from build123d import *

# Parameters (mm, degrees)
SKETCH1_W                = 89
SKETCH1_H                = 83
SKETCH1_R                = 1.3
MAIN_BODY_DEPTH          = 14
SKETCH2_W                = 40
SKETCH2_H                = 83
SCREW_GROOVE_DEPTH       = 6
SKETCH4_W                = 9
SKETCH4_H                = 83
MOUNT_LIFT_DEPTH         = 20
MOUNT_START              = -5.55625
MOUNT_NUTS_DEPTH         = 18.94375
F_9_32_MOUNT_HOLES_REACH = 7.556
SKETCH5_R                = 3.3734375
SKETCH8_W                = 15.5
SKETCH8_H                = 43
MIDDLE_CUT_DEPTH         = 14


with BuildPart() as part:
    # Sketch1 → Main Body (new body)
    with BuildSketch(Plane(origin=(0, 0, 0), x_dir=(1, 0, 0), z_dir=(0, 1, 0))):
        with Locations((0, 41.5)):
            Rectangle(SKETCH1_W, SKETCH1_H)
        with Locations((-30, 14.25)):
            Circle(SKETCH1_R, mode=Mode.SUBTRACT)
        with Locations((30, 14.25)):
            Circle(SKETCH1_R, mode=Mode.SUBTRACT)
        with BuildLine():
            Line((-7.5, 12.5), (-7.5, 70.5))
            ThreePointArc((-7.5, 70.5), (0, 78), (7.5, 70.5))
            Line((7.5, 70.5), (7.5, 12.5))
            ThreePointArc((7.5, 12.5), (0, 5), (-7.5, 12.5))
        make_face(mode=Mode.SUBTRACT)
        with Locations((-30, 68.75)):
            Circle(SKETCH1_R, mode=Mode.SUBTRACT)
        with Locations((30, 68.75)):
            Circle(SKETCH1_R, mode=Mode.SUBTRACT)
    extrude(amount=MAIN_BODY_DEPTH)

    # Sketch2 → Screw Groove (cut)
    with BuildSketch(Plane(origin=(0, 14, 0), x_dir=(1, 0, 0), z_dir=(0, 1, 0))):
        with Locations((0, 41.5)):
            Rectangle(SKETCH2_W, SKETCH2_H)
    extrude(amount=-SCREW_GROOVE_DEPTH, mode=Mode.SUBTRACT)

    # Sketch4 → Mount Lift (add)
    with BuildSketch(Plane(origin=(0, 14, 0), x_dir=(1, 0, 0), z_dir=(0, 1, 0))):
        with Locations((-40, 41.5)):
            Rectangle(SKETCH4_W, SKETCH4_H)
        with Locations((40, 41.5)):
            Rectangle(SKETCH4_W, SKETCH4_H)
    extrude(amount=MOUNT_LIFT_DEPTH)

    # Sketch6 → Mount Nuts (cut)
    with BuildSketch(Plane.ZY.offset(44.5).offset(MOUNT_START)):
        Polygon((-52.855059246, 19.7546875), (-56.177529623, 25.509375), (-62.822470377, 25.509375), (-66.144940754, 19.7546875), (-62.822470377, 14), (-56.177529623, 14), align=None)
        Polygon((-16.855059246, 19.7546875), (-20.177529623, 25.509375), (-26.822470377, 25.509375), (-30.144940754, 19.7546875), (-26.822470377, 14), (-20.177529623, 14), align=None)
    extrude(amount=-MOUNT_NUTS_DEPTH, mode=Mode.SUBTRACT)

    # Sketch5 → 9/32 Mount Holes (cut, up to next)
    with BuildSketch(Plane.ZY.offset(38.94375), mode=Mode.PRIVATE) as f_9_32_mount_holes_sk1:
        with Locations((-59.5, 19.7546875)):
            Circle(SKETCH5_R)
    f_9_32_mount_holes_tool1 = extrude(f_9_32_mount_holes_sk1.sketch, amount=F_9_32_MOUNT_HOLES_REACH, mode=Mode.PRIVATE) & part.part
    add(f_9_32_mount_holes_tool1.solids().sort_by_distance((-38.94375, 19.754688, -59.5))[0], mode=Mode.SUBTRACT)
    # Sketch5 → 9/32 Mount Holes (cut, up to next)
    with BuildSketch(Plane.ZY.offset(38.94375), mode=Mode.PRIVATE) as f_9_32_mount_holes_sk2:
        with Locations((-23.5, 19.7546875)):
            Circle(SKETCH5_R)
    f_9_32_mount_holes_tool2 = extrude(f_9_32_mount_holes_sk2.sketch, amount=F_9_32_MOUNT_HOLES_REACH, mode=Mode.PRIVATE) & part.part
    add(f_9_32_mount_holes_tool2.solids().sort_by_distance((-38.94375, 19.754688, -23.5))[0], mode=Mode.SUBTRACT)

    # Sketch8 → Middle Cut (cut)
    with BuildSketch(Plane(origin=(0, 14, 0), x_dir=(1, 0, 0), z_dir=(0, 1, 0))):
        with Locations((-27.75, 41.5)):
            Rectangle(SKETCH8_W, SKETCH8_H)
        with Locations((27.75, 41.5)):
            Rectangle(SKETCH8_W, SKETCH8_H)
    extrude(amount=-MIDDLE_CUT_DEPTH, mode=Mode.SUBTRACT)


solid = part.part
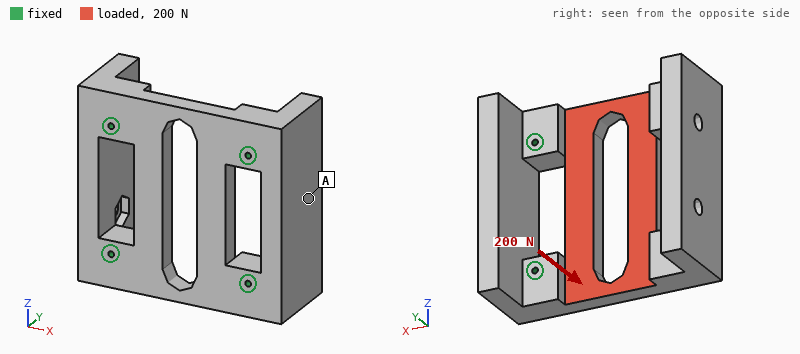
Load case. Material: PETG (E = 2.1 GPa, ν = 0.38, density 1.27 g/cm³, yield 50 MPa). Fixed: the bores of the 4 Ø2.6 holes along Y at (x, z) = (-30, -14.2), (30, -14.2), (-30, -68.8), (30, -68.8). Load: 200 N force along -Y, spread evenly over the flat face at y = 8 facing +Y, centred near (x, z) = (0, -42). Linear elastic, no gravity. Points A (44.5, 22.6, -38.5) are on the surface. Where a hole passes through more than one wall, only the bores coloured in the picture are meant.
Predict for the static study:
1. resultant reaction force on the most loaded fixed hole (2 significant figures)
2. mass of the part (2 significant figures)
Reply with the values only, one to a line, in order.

51 N
110 g
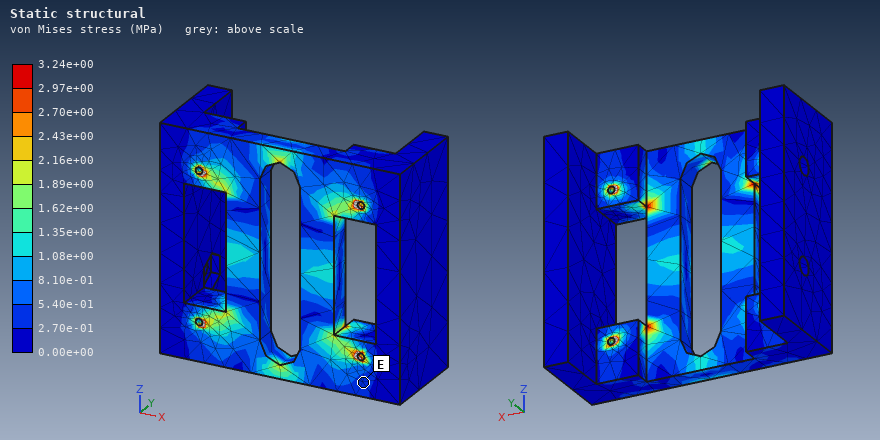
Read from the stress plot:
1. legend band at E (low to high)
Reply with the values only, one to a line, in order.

2.70e-01 to 5.40e-01 MPa
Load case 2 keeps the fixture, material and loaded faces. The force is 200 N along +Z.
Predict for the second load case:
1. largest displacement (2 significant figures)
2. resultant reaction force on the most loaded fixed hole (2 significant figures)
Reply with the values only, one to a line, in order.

19 µm
53 N
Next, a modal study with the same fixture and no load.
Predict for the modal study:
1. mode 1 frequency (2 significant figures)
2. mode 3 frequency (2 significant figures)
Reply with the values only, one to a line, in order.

1500 Hz
2200 Hz
